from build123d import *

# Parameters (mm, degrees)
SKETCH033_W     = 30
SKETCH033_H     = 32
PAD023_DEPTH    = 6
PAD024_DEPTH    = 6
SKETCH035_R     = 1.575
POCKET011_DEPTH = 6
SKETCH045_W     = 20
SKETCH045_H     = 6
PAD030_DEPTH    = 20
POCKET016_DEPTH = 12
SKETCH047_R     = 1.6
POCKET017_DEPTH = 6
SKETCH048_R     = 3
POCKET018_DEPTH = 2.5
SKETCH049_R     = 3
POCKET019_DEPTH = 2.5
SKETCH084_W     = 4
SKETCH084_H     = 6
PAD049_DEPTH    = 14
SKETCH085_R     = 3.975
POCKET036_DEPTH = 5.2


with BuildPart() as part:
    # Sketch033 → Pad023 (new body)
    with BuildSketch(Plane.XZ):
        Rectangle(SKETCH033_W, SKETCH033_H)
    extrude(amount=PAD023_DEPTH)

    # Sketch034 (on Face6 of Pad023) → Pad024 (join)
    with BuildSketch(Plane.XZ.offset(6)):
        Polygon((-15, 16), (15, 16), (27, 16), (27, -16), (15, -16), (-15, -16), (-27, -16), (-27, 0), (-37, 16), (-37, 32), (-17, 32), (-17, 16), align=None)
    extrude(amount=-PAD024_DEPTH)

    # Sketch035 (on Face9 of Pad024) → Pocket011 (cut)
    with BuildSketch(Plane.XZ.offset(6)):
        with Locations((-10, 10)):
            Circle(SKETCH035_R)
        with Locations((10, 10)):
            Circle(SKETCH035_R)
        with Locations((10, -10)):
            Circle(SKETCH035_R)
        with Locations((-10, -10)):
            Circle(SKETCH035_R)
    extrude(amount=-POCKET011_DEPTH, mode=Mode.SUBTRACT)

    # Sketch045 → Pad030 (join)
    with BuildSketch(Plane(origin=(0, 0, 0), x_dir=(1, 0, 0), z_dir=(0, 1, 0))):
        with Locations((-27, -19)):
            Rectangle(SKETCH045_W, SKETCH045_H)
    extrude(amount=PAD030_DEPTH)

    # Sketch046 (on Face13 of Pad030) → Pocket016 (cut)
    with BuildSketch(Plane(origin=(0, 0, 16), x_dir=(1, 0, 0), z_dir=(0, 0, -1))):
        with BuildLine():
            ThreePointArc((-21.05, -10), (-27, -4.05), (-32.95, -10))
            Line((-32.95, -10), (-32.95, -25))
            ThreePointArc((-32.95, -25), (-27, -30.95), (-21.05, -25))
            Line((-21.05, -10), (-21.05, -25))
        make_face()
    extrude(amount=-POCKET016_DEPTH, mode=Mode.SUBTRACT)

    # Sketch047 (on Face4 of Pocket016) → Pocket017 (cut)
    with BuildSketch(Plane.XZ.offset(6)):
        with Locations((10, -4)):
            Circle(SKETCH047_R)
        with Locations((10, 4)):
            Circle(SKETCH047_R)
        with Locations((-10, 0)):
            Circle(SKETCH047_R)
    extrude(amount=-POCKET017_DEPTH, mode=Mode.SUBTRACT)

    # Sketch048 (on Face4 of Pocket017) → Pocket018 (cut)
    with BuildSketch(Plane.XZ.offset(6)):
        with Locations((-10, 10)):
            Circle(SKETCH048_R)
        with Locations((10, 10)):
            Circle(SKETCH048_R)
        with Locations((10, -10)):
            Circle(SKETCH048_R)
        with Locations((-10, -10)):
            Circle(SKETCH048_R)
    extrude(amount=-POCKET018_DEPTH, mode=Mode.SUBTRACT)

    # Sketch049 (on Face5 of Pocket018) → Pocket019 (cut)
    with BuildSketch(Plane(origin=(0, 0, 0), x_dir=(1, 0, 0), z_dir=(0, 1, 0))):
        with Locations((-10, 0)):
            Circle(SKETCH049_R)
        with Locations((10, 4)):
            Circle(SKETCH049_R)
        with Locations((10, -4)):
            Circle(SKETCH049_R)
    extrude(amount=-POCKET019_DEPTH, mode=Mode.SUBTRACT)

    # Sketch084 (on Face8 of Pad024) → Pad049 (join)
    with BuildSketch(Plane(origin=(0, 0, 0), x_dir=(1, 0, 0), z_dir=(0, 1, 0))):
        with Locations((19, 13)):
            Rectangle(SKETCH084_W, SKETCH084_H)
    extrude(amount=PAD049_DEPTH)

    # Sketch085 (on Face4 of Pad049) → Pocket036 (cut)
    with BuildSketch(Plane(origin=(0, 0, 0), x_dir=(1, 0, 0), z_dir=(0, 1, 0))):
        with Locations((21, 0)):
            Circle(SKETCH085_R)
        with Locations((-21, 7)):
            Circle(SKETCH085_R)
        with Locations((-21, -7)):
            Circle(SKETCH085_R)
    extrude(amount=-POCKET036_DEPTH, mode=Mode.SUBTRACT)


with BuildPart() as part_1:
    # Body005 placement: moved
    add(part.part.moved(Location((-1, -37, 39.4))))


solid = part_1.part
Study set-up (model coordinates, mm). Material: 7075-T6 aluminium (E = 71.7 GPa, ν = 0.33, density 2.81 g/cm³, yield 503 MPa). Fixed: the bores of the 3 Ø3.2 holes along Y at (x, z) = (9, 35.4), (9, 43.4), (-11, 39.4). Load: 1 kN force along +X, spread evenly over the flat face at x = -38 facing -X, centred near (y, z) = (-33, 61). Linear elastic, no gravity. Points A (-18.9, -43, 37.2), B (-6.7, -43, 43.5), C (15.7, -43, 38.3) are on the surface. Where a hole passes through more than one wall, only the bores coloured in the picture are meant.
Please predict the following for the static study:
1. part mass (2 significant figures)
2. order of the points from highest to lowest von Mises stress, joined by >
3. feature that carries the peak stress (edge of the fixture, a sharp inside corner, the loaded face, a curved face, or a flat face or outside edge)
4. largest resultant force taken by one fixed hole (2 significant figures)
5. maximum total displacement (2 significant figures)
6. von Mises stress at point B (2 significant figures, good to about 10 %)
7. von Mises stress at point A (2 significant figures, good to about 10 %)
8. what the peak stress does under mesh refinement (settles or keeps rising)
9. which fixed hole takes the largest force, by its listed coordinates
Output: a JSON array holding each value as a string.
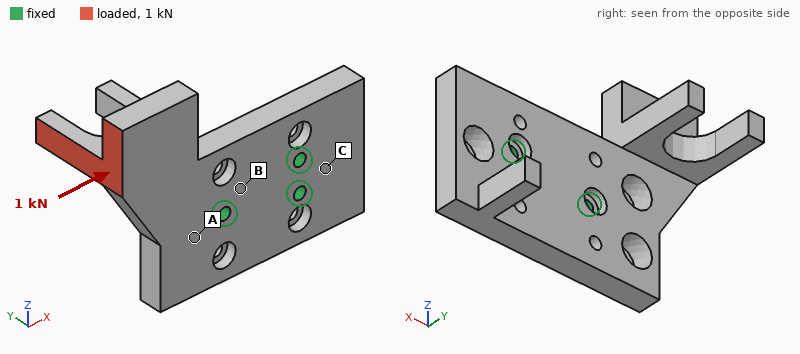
["37 g", "A > B > C", "a sharp inside corner", "1.0 kN", "0.31 mm", "18 MPa", "54 MPa", "keeps rising", "(9, 43.4)"]
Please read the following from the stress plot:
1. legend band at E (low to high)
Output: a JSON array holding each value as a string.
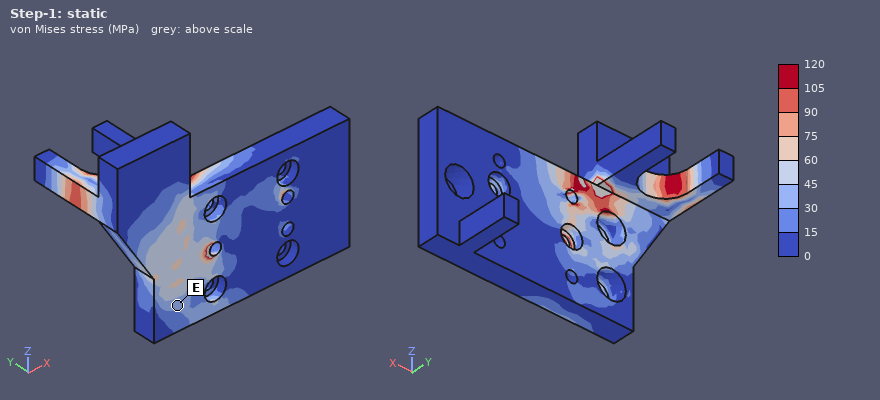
["30 to 45 MPa"]
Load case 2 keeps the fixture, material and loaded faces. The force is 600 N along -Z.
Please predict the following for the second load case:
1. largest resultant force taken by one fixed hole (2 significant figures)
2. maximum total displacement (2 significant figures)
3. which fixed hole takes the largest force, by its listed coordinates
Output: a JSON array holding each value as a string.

["1.1 kN", "0.25 mm", "(-11, 39.4)"]
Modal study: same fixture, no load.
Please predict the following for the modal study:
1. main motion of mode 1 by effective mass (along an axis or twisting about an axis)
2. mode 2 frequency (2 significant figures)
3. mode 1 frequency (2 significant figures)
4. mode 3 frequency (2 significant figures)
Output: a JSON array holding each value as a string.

["along Y", "4800 Hz", "2200 Hz", "7700 Hz"]
